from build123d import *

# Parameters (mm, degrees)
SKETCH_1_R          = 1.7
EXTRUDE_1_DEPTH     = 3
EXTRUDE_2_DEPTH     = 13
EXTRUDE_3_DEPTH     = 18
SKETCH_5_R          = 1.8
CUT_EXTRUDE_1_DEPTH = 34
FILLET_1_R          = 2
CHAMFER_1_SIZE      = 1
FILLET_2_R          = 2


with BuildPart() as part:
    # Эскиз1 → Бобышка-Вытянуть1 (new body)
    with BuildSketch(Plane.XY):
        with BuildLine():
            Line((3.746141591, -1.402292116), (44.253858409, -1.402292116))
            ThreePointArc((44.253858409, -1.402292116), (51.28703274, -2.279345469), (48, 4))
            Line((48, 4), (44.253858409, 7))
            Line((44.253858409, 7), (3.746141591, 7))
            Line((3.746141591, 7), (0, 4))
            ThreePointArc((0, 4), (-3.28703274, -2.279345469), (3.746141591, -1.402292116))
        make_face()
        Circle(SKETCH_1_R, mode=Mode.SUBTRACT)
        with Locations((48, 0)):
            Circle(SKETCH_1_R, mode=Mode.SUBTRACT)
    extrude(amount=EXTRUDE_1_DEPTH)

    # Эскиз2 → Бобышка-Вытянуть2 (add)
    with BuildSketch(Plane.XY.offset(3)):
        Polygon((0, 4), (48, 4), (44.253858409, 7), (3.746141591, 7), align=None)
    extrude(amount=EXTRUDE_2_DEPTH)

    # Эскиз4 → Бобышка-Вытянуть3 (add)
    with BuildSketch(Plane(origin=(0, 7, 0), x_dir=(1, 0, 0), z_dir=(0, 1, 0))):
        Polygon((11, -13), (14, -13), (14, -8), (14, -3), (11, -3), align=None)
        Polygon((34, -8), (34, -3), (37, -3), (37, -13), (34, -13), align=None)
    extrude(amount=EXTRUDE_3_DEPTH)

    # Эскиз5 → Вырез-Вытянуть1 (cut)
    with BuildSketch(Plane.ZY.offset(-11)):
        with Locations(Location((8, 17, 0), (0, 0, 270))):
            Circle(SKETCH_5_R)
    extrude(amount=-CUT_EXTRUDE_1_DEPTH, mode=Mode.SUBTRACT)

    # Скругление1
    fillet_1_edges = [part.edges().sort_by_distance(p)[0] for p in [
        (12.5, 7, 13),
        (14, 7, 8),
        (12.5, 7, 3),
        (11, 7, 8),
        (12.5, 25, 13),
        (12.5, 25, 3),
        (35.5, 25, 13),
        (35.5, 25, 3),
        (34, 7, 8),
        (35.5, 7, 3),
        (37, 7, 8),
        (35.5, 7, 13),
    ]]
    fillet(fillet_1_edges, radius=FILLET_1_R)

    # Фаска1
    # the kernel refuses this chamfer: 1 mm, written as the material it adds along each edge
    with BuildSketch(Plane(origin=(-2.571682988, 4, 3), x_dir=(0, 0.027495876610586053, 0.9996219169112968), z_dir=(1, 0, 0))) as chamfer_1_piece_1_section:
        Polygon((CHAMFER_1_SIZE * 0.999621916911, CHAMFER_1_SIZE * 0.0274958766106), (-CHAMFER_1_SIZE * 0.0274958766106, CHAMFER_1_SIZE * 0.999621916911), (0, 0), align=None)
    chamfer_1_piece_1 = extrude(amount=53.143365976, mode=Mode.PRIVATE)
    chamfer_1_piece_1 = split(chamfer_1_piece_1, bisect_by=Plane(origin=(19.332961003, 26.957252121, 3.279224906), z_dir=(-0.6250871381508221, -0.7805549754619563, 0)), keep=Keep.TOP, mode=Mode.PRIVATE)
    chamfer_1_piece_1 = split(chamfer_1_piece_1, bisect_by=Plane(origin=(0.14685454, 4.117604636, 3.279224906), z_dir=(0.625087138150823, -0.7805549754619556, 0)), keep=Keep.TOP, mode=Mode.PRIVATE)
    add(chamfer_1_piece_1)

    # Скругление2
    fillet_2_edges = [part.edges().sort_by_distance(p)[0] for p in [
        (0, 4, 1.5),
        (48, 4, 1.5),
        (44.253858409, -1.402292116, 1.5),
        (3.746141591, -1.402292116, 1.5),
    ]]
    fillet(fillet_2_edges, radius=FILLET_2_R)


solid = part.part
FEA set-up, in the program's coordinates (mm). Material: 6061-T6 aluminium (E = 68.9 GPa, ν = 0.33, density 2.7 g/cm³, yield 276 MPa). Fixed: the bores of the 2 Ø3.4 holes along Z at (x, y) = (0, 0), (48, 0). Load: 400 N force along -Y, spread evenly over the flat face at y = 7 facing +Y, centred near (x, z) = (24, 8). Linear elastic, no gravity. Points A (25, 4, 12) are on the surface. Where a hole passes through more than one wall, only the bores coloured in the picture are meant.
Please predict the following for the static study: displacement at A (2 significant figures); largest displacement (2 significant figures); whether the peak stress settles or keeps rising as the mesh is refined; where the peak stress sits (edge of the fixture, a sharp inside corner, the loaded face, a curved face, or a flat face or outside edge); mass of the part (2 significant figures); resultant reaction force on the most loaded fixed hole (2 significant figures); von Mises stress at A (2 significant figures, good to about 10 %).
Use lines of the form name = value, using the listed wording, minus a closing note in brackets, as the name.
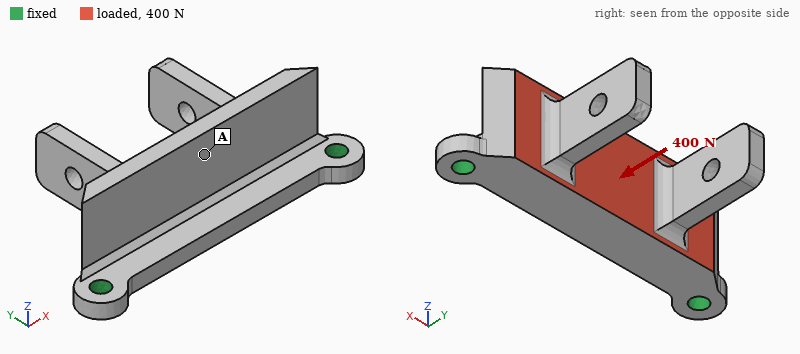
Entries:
displacement at A = 0.090 mm
largest displacement = 0.17 mm
whether the peak stress settles or keeps rising as the mesh is refined = keeps rising
where the peak stress sits = edge of the fixture
mass of the part = 11 g
resultant reaction force on the most loaded fixed hole = 270 N
von Mises stress at A = 20 MPa
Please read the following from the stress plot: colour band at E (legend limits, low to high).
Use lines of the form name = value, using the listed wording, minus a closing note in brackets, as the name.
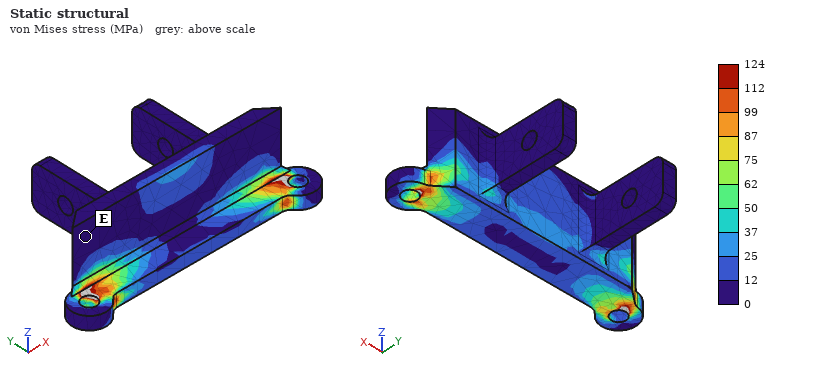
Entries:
colour band at E = 0 to 12 MPa
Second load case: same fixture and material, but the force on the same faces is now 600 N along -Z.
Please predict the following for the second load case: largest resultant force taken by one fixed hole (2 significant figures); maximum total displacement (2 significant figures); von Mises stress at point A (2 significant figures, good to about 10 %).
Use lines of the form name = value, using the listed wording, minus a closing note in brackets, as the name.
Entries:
largest resultant force taken by one fixed hole = 320 N
maximum total displacement = 0.16 mm
von Mises stress at point A = 19 MPa
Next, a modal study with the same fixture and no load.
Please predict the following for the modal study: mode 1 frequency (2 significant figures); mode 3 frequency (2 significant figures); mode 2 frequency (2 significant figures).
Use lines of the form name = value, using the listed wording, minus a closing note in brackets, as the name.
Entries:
mode 1 frequency = 2900 Hz
mode 3 frequency = 6500 Hz
mode 2 frequency = 6300 Hz
